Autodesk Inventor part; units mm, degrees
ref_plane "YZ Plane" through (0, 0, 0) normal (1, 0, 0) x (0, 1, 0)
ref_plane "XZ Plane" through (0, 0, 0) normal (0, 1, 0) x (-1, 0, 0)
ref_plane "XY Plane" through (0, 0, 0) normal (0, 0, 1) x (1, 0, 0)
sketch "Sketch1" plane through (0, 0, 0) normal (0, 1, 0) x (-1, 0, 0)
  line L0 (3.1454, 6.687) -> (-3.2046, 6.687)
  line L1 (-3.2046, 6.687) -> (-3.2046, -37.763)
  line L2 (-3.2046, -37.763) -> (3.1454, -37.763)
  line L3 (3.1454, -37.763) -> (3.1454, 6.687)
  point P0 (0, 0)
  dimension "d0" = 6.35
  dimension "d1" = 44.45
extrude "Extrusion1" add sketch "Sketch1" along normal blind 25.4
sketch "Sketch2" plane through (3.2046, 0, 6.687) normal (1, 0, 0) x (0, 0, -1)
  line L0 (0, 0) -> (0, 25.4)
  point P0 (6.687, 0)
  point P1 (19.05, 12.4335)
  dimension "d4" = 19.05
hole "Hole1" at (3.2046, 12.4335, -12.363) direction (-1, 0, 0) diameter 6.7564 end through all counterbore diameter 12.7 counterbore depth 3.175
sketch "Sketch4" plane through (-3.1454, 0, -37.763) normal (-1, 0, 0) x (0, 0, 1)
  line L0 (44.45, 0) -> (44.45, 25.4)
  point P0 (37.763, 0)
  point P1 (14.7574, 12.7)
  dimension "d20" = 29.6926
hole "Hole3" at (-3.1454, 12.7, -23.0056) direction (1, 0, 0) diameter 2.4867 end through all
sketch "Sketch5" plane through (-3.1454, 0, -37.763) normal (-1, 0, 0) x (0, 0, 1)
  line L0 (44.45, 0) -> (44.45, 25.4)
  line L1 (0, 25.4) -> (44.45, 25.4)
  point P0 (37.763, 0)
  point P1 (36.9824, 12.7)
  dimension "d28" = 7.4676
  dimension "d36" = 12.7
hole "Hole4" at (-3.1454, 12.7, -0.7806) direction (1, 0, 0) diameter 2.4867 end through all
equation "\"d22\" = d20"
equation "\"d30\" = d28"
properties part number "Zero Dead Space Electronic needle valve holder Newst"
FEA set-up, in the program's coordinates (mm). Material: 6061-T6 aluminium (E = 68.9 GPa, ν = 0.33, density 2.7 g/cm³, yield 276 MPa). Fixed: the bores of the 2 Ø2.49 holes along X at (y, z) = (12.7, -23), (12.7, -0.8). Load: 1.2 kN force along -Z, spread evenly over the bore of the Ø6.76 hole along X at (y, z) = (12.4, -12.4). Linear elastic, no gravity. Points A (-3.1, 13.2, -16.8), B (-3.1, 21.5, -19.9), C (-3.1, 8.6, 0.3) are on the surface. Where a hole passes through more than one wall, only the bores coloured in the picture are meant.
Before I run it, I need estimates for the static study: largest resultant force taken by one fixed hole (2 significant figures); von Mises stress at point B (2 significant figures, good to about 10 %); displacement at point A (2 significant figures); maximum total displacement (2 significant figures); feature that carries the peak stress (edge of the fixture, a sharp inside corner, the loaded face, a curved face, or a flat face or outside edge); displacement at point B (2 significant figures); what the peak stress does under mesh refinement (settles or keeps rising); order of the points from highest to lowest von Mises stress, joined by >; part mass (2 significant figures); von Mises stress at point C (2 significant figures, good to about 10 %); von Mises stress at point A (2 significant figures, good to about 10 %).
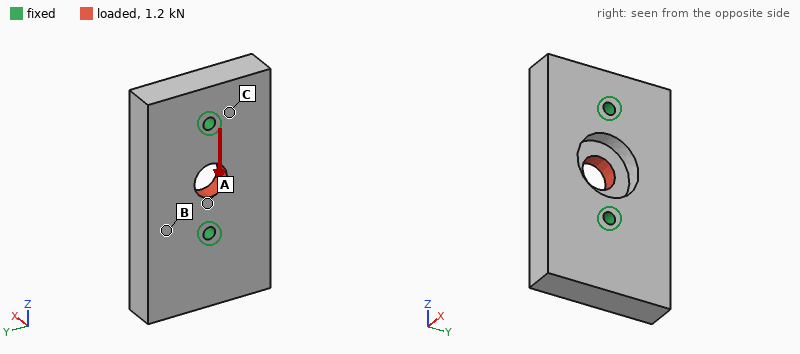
630 N
2.5 MPa
1.7 µm
2.4 µm
edge of the fixture
0.94 µm
keeps rising
A > C > B
18 g
5.4 MPa
20 MPa
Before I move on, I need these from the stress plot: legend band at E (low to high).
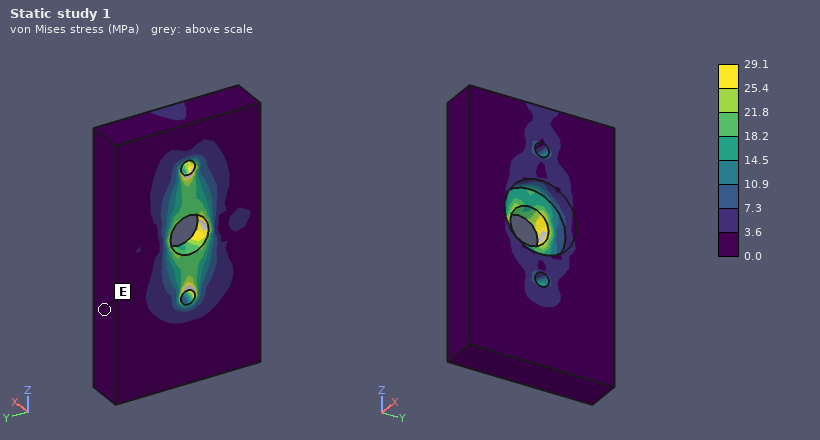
0.0 to 3.6 MPa
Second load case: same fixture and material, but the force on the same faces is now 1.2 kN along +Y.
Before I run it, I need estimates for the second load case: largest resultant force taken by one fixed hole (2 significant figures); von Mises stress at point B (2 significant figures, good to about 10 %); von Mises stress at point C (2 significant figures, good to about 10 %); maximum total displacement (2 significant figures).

620 N
8.7 MPa
8.6 MPa
4.2 µm
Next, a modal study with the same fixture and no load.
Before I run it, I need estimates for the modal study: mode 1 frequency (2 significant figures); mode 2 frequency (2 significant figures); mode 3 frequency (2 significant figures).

16 kHz
16 kHz
21 kHz
